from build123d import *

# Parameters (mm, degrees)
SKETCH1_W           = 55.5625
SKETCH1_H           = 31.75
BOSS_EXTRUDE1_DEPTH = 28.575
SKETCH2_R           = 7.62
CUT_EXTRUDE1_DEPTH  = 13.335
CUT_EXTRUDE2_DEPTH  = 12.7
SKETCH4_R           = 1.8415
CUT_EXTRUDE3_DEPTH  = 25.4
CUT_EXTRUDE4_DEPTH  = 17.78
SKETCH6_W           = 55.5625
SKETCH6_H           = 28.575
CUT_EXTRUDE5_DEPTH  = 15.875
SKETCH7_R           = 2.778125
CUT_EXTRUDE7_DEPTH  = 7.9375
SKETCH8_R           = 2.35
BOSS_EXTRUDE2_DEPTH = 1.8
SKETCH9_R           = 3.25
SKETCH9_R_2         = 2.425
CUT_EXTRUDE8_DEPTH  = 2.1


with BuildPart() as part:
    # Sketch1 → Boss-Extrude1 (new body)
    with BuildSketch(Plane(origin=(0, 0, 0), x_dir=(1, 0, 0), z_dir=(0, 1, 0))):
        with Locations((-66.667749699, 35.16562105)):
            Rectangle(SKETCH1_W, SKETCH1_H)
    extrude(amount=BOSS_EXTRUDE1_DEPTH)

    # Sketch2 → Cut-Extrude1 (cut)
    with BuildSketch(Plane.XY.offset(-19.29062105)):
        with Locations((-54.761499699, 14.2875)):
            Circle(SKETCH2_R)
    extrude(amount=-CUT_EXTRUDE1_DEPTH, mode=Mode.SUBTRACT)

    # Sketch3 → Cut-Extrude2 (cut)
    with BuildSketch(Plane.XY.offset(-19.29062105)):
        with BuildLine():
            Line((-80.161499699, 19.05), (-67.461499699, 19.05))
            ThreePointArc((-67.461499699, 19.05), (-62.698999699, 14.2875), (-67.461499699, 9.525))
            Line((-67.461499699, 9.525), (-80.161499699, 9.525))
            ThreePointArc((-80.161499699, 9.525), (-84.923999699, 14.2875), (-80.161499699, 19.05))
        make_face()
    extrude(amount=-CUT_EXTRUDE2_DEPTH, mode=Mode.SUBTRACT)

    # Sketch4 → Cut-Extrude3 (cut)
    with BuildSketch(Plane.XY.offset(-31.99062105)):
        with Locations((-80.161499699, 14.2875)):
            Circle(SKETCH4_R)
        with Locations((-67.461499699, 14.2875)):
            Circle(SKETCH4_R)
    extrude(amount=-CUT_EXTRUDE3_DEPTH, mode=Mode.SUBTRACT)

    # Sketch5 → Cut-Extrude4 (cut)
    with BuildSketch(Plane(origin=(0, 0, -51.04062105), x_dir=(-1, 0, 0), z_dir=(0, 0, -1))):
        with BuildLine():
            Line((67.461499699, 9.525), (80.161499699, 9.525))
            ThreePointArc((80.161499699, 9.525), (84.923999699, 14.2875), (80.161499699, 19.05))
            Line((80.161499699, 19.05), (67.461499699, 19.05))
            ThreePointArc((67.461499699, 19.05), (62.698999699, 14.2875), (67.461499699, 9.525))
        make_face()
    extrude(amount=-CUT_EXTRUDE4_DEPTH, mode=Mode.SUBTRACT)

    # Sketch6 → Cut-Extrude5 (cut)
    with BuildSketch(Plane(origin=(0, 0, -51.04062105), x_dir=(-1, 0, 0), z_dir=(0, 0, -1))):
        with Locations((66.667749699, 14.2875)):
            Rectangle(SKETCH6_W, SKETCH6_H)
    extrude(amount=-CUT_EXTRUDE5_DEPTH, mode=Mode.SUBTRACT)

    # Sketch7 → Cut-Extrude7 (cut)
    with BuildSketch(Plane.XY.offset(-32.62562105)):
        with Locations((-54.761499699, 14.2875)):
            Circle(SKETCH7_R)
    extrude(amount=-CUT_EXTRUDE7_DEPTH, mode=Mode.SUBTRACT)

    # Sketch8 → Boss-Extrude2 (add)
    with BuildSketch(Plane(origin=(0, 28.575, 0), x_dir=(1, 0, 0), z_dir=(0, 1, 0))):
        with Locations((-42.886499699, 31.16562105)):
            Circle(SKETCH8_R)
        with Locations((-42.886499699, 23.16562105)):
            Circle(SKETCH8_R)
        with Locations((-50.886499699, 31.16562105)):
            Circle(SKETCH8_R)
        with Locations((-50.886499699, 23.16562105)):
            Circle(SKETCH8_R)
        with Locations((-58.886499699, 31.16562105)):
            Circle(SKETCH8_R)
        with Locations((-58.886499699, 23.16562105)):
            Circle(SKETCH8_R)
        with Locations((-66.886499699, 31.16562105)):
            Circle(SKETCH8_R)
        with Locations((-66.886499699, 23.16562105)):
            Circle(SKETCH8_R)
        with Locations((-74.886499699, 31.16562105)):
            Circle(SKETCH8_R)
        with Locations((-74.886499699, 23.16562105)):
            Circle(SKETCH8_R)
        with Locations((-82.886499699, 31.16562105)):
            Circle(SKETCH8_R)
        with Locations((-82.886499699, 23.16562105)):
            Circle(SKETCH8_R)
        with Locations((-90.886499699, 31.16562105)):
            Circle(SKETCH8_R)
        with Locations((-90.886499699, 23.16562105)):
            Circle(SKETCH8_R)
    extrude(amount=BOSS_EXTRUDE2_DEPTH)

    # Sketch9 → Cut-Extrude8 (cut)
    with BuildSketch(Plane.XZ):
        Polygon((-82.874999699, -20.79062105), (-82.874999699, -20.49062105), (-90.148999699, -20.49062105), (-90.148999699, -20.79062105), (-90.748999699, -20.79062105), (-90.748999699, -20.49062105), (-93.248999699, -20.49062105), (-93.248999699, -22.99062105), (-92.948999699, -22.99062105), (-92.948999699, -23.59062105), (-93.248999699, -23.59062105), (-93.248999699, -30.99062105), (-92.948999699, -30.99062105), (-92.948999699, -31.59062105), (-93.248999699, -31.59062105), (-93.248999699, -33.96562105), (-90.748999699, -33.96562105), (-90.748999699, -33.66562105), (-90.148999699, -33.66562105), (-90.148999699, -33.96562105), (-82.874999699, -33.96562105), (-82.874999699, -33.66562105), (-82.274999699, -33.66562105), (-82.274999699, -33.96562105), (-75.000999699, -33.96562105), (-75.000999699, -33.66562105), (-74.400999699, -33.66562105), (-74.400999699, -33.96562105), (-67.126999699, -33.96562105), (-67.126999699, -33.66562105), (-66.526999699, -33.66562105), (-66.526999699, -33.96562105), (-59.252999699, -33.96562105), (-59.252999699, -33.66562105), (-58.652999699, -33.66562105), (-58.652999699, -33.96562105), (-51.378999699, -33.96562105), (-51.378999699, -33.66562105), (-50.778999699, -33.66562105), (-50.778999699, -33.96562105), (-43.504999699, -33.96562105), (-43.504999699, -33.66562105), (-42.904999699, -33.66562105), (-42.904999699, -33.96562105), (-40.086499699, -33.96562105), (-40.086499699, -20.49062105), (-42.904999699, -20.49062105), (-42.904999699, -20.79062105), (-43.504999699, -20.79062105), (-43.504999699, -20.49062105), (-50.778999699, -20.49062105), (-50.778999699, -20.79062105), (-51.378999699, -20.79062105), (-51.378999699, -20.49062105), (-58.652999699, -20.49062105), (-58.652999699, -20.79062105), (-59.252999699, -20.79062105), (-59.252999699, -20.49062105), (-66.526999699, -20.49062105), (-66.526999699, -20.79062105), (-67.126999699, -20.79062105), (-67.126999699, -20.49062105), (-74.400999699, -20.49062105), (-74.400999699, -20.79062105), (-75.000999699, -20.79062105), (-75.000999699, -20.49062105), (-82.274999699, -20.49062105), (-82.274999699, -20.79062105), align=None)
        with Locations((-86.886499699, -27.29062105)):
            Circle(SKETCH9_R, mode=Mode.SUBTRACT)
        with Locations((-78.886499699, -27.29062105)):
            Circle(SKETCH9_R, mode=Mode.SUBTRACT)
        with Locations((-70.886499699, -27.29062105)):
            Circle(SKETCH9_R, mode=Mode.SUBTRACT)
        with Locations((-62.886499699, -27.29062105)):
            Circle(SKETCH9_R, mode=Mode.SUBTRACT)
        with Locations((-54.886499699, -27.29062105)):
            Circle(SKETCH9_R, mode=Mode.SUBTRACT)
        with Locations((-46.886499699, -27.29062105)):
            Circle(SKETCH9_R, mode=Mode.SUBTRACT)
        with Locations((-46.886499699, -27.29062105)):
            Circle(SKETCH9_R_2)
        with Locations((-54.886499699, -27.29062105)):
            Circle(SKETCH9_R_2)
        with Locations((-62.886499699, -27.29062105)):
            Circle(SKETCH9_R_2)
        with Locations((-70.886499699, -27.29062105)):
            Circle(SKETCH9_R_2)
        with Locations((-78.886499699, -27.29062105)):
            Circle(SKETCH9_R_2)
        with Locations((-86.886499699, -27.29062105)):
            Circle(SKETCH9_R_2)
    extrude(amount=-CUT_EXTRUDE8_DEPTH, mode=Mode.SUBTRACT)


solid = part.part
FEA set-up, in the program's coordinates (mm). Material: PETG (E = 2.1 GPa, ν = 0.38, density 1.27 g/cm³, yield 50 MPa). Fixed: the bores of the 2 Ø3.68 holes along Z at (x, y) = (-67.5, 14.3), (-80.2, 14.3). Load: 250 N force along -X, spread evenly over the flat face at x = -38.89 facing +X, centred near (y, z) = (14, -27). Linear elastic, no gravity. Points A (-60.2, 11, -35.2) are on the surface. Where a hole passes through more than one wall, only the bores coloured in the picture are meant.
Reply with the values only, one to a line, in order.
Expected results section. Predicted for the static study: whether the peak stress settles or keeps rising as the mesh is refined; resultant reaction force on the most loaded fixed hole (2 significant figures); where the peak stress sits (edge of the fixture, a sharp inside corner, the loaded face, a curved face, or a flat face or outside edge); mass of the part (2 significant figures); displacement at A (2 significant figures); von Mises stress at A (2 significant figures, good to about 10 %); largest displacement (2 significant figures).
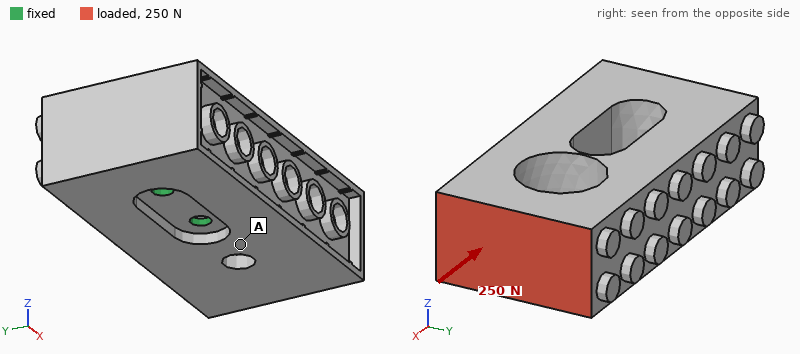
keeps rising
160 N
edge of the fixture
24 g
0.099 mm
3.0 MPa
0.32 mm
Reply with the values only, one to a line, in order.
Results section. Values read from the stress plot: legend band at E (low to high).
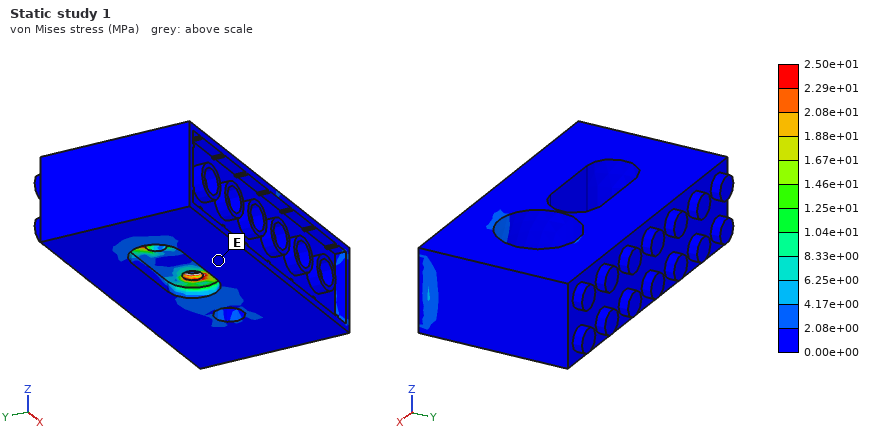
0.00e+00 to 2.08e+00 MPa
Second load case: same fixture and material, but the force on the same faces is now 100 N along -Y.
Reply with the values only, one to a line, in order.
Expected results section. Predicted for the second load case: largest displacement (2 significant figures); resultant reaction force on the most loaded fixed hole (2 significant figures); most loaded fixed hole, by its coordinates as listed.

0.68 mm
280 N
(-67.5, 14.3)
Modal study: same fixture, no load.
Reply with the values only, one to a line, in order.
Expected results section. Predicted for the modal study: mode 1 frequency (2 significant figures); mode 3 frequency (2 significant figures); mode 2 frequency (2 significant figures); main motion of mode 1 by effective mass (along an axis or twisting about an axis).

440 Hz
1200 Hz
660 Hz
along Y
